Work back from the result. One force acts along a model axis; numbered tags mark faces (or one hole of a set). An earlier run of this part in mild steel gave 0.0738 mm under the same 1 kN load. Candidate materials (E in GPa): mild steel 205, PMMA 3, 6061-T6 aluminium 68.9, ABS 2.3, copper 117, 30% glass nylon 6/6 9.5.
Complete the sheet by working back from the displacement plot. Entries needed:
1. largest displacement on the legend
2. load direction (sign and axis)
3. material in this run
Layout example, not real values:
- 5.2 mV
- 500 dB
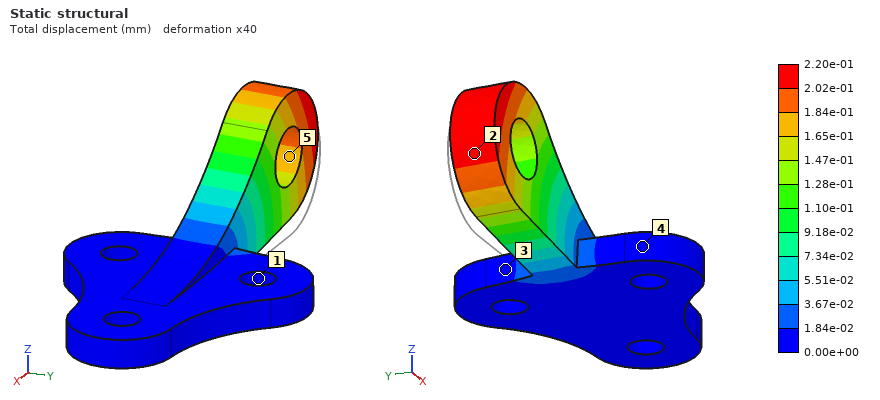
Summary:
- 2.20e-01 mm
- +Z
- 6061-T6 aluminium
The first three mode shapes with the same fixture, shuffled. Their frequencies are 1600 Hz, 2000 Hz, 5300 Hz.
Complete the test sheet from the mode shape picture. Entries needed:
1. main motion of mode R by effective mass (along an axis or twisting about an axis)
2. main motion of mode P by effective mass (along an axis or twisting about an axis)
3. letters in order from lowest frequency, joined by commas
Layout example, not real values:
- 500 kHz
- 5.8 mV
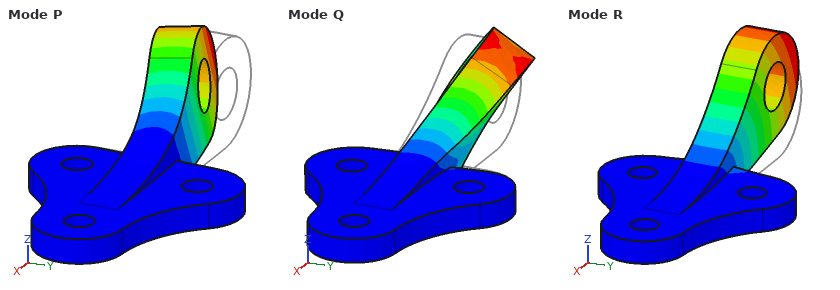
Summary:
- along Z
- along Y
- R, P, Q
